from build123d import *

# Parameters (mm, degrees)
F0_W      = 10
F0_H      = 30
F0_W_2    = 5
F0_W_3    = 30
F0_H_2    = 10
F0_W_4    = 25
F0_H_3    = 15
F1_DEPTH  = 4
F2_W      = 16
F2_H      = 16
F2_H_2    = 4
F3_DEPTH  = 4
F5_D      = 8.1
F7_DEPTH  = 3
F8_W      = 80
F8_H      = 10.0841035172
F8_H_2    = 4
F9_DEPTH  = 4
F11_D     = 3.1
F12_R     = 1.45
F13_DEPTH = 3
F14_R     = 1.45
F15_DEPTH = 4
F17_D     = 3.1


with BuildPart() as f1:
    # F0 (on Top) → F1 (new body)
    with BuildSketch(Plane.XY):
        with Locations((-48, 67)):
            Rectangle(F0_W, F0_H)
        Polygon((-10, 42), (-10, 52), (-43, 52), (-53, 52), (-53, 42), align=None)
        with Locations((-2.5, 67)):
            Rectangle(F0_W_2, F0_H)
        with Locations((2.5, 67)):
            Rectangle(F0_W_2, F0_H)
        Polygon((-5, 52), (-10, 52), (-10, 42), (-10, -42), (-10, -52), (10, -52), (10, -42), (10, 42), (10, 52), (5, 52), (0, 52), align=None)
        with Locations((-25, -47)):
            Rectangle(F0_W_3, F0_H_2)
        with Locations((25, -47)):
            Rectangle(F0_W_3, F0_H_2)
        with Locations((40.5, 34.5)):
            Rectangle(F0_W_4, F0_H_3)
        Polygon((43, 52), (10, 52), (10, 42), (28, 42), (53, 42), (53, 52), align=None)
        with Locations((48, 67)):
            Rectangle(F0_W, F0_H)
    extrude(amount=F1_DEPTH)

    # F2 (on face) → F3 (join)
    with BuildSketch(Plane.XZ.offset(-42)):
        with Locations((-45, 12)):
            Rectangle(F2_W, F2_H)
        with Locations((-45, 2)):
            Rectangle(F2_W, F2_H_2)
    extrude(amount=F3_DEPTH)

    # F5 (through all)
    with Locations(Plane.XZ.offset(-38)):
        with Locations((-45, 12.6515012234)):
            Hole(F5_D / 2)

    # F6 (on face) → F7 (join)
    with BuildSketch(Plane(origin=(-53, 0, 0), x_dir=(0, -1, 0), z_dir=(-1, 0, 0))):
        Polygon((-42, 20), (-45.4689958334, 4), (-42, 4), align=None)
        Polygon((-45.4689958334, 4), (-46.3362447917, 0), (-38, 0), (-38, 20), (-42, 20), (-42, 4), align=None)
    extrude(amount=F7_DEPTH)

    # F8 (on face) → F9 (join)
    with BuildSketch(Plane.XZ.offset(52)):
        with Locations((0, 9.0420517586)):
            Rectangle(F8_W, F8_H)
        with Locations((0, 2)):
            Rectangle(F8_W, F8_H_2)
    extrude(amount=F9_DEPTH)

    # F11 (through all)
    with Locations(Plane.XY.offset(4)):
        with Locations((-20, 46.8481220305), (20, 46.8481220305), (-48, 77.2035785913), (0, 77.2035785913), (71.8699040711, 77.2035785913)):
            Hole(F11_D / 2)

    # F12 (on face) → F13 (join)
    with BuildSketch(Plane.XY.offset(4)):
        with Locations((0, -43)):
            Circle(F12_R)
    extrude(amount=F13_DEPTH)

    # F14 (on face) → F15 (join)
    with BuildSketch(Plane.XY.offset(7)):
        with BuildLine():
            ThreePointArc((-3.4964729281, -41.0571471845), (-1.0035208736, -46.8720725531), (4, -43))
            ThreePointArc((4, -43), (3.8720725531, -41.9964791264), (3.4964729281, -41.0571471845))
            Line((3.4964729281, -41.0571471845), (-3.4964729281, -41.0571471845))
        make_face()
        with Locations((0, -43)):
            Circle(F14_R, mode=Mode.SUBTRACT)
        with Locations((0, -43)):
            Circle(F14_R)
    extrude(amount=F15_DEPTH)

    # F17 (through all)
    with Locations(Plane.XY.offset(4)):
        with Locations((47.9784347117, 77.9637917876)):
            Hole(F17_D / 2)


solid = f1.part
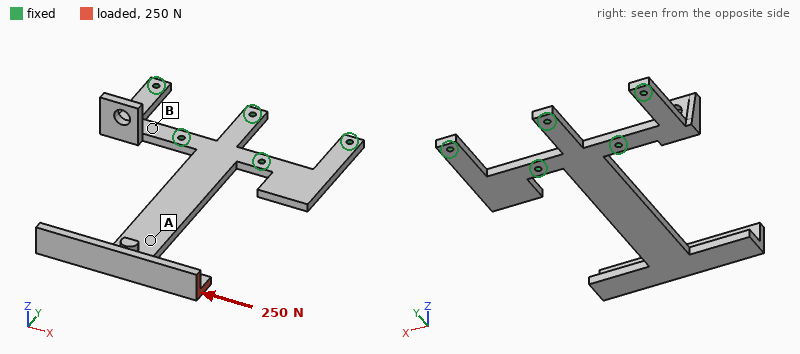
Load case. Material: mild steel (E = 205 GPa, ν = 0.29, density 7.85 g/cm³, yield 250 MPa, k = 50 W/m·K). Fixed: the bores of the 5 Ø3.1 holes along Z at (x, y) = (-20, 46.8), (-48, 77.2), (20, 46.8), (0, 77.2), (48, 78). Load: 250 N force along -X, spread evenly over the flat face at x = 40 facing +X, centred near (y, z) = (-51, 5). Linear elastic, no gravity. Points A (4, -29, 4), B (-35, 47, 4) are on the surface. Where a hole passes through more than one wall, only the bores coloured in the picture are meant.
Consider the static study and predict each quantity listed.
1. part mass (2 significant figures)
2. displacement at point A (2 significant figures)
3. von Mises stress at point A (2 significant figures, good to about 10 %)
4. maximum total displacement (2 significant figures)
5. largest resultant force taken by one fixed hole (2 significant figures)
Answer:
200 g
0.12 mm
22 MPa
0.25 mm
700 N
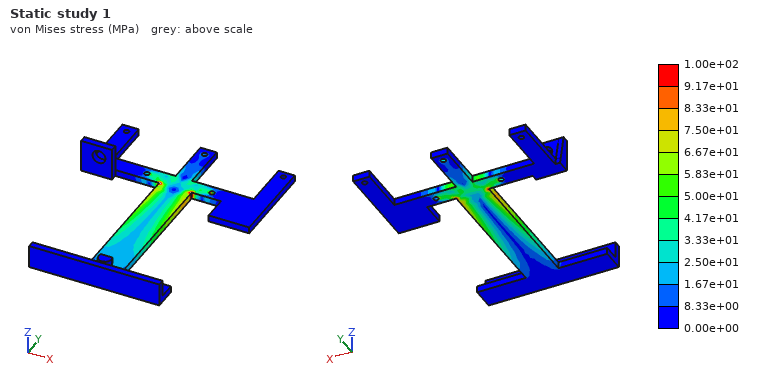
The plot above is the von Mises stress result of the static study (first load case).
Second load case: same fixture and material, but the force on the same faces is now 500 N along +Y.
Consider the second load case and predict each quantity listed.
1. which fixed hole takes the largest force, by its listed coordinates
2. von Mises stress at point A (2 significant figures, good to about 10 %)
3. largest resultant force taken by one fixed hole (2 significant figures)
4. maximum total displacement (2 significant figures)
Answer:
(20, 46.8)
61 MPa
680 N
0.55 mm
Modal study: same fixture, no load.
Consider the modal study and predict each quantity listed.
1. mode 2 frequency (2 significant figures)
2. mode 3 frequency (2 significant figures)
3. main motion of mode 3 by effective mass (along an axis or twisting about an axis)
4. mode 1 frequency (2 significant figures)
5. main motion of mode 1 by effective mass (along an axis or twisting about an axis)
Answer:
490 Hz
690 Hz
along X
150 Hz
along Z
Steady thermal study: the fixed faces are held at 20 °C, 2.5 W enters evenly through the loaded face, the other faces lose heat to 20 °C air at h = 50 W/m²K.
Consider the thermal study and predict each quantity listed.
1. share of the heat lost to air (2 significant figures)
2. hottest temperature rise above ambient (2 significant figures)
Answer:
96 %
20 K
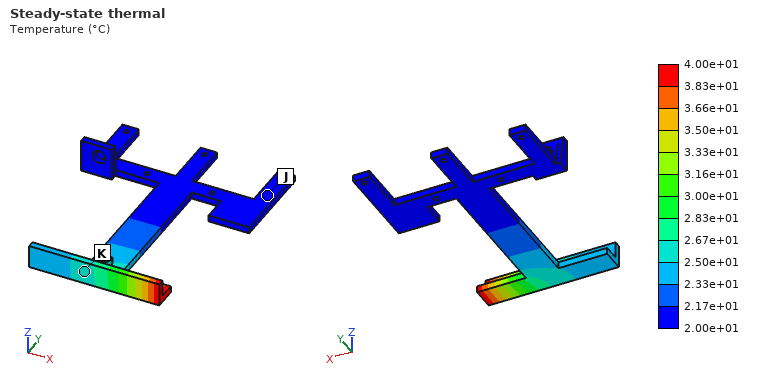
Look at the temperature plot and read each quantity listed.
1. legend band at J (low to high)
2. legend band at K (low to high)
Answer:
2.00e+01 to 2.17e+01 °C
2.50e+01 to 2.67e+01 °C
